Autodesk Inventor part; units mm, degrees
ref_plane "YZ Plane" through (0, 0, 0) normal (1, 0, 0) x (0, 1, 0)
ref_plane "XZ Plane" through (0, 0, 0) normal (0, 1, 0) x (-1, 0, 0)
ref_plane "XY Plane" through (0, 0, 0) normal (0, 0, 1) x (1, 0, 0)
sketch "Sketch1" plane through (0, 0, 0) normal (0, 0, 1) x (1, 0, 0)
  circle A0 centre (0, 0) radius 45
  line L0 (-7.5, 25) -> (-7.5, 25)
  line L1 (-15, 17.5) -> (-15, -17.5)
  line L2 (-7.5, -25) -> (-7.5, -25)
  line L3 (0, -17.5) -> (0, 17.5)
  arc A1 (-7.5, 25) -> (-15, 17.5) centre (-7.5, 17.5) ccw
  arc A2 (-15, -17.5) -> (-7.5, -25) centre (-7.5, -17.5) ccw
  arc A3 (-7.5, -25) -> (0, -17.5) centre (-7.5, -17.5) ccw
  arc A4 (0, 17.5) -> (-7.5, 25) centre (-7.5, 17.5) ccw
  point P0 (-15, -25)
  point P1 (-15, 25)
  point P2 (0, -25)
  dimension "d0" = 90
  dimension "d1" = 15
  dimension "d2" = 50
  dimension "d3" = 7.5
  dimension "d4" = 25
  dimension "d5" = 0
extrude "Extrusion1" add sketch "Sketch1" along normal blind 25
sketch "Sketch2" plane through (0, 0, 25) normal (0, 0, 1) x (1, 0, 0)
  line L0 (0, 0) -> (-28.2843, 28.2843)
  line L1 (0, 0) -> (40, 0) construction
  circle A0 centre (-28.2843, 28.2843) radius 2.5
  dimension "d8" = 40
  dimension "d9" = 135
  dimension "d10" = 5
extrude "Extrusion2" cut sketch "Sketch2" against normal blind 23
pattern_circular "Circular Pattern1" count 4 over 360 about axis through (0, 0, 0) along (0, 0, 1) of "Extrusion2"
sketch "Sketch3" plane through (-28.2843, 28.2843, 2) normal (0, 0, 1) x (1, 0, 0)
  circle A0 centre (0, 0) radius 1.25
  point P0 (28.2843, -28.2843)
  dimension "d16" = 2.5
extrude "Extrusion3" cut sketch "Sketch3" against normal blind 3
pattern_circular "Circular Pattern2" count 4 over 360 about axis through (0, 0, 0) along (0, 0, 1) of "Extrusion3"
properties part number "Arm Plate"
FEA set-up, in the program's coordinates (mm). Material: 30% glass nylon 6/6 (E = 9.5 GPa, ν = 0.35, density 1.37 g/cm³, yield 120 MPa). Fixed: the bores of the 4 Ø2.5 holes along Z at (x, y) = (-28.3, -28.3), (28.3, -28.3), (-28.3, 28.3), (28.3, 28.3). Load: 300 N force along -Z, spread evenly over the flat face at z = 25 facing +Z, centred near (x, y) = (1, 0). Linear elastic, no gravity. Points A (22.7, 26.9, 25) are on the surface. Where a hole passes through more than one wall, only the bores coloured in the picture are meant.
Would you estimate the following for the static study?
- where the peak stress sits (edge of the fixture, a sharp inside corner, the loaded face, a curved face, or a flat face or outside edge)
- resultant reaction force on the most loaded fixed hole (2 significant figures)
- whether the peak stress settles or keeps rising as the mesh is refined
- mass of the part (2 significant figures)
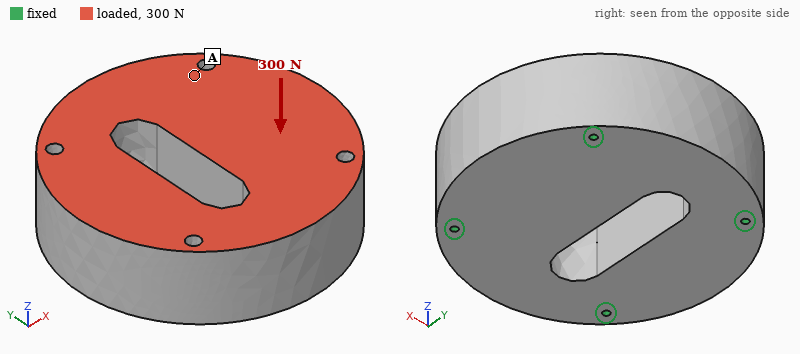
edge of the fixture
80 N
keeps rising
190 g
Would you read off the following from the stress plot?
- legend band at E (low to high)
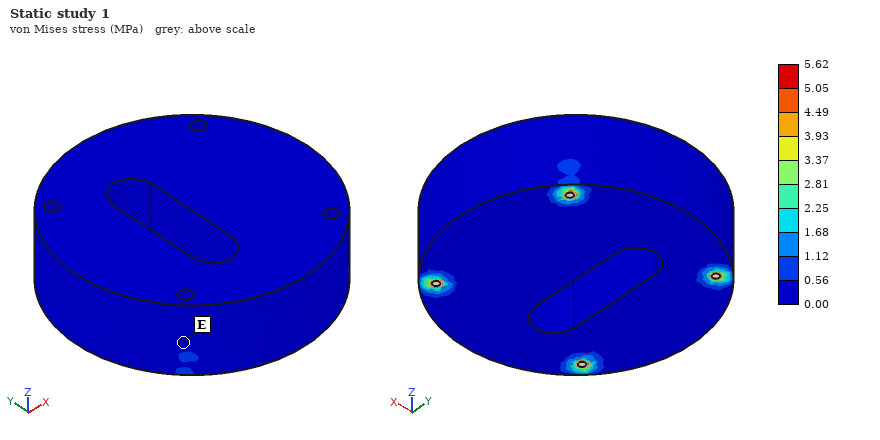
0.00 to 0.56 MPa
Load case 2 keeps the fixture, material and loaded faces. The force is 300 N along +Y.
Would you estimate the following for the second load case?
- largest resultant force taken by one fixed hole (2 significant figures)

100 N
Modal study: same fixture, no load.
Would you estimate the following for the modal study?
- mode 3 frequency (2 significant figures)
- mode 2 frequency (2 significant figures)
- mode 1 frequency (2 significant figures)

3400 Hz
3300 Hz
3200 Hz
